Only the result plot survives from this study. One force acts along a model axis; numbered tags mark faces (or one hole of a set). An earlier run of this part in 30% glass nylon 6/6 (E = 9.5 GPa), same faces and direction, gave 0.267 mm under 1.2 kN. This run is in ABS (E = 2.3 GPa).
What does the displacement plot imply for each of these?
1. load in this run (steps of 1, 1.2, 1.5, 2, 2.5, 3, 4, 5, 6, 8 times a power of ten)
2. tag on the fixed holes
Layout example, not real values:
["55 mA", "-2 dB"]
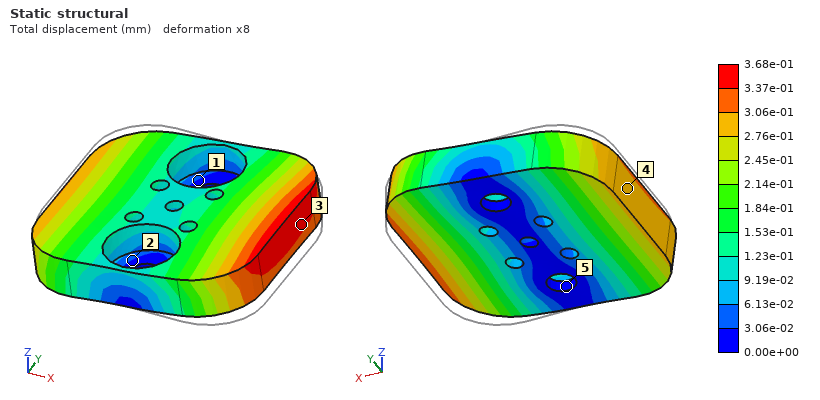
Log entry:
["400 N", "5"]
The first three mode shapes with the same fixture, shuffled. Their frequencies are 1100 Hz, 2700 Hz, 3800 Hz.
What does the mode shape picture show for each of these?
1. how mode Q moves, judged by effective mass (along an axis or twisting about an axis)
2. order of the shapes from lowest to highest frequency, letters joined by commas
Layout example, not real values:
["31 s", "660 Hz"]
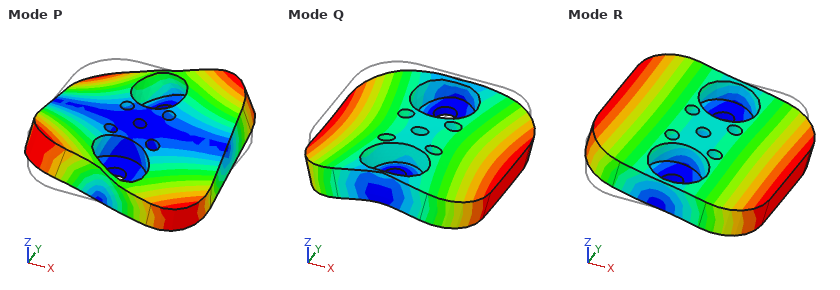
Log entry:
["along Z", "R, Q, P"]
